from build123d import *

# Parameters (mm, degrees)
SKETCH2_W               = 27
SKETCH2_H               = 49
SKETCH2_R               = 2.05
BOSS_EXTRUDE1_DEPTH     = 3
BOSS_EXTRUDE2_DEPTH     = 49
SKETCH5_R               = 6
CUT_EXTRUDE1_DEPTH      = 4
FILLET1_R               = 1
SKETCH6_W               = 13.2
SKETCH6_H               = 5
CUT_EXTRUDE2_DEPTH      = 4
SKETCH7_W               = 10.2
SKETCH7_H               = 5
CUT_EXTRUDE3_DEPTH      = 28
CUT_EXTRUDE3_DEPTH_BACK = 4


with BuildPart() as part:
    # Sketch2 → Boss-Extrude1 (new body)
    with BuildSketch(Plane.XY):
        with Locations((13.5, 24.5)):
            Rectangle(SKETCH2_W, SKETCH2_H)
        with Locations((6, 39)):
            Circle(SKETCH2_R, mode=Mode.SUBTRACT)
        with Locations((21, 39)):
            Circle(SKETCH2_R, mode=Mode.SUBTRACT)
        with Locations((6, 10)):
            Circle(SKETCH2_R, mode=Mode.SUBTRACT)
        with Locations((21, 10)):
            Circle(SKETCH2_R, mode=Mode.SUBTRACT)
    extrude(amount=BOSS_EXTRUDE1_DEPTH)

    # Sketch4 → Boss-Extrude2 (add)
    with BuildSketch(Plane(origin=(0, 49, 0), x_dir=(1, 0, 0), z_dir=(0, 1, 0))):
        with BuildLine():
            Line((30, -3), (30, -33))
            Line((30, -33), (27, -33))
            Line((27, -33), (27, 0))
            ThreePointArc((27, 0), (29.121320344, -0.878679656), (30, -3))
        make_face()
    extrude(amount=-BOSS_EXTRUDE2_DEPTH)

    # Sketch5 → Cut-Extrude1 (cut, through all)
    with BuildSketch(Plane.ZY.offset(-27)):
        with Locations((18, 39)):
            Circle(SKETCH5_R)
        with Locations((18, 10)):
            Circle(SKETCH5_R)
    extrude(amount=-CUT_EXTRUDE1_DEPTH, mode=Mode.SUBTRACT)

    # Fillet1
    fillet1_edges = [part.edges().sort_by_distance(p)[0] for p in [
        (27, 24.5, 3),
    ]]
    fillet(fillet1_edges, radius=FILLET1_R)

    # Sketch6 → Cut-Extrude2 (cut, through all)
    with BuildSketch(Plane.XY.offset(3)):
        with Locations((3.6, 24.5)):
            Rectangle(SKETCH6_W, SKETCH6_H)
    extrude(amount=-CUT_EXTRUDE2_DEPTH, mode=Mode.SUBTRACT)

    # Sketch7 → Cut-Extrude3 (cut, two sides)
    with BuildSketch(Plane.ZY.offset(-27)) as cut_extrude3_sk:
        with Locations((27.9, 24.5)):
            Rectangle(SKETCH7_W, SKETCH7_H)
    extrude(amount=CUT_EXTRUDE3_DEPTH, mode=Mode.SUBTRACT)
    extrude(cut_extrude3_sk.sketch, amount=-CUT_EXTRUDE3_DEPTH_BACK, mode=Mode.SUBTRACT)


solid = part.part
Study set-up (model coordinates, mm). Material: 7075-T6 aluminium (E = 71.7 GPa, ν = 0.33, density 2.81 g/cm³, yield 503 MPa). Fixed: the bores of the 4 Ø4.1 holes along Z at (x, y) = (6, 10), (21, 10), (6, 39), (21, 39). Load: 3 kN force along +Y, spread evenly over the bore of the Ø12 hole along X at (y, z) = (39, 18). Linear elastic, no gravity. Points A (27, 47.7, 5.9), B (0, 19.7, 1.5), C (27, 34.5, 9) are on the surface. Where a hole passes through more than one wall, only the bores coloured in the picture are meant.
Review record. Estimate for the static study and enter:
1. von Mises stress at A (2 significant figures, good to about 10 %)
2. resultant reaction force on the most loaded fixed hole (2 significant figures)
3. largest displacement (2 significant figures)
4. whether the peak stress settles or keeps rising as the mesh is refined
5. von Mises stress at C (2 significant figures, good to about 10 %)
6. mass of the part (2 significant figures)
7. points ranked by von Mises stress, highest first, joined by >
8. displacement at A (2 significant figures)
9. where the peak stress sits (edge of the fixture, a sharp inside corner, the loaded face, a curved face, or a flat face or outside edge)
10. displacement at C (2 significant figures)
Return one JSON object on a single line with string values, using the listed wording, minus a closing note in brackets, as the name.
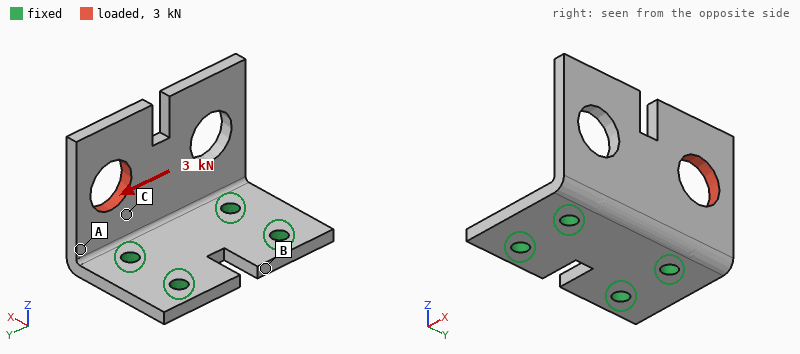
{"von Mises stress at A": "86 MPa", "resultant reaction force on the most loaded fixed hole": "2.3 kN", "largest displacement": "0.25 mm", "whether the peak stress settles or keeps rising as the mesh is refined": "keeps rising", "von Mises stress at C": "140 MPa", "mass of the part": "21 g", "points ranked by von Mises stress, highest first, joined by >": "C > A > B", "displacement at A": "0.093 mm", "where the peak stress sits": "edge of the fixture", "displacement at C": "0.061 mm"}
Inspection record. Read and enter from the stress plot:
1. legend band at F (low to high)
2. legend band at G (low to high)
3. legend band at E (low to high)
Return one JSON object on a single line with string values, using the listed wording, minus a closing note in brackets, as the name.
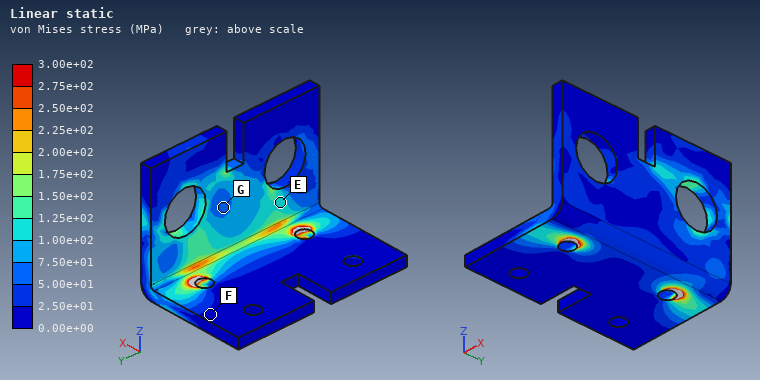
{"legend band at F": "0.00e+00 to 2.50e+01 MPa", "legend band at G": "5.00e+01 to 7.50e+01 MPa", "legend band at E": "1.00e+02 to 1.25e+02 MPa"}
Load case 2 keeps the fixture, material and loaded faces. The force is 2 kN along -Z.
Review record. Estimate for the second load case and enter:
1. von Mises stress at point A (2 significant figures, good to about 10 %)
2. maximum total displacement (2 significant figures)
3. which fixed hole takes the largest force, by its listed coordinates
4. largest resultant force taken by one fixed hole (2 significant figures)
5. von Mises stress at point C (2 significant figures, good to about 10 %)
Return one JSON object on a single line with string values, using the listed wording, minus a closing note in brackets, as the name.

{"von Mises stress at point A": "57 MPa", "maximum total displacement": "0.35 mm", "which fixed hole takes the largest force, by its listed coordinates": "(21, 39)", "largest resultant force taken by one fixed hole": "2.1 kN", "von Mises stress at point C": "75 MPa"}
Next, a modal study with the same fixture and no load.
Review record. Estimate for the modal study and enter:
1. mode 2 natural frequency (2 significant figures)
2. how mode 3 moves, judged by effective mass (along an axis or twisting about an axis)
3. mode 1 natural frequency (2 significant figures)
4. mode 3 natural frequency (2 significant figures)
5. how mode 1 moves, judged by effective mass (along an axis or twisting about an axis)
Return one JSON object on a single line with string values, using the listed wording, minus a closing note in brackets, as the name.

{"mode 2 natural frequency": "3200 Hz", "how mode 3 moves, judged by effective mass": "along Y", "mode 1 natural frequency": "2000 Hz", "mode 3 natural frequency": "7500 Hz", "how mode 1 moves, judged by effective mass": "along X"}
